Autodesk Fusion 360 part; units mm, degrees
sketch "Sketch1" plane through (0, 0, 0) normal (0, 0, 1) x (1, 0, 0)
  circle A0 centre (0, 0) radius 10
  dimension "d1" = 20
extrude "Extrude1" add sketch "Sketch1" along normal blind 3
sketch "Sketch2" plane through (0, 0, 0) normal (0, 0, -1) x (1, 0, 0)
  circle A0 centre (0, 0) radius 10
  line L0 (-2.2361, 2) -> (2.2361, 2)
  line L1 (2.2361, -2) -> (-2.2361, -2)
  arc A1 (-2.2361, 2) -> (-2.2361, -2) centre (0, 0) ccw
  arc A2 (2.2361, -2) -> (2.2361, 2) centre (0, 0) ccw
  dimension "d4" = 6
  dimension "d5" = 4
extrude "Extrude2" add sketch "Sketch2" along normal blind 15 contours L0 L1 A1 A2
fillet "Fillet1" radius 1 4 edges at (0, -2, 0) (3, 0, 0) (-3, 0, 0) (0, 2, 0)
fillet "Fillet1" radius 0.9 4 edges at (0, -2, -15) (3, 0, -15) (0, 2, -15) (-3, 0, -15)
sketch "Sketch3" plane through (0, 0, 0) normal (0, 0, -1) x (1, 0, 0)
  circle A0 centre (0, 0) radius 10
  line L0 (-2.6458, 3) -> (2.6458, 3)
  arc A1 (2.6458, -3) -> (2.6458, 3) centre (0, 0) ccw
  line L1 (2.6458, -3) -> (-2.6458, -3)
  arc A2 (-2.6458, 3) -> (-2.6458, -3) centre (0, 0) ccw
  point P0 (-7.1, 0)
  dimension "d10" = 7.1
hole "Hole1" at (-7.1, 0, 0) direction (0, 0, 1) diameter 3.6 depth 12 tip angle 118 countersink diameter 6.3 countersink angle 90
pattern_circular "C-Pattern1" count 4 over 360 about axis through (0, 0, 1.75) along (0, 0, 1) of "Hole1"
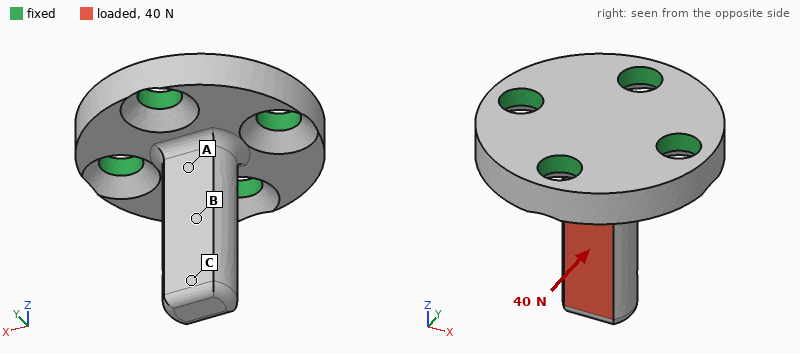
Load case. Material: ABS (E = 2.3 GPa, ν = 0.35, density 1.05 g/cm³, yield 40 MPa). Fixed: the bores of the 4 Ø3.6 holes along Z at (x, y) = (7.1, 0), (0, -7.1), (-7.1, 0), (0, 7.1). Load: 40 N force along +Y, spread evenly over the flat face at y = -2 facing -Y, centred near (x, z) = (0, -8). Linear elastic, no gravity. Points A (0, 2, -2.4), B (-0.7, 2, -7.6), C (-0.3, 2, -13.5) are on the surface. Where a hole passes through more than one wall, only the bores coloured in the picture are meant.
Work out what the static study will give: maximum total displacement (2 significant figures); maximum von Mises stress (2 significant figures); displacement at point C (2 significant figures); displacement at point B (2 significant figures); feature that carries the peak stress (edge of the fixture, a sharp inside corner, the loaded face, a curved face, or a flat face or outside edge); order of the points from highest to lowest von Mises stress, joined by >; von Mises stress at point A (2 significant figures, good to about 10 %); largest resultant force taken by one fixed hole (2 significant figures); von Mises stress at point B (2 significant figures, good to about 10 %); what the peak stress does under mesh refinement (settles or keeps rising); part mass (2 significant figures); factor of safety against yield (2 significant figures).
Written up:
0.34 mm
30 MPa
0.31 mm
0.15 mm
a curved face
A > B > C
14 MPa
37 N
4.9 MPa
settles
1.2 g
1.3
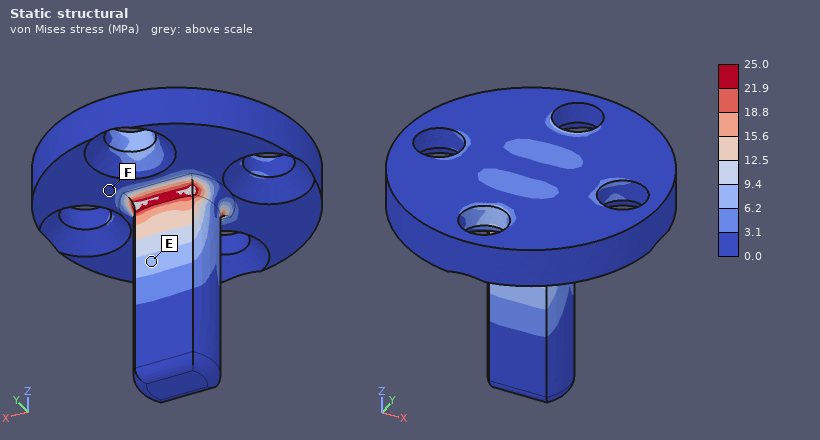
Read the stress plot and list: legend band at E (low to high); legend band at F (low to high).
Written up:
6.2 to 9.4 MPa
0.0 to 3.1 MPa
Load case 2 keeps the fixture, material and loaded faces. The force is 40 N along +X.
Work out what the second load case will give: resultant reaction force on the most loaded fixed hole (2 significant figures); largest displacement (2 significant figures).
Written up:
38 N
0.21 mm
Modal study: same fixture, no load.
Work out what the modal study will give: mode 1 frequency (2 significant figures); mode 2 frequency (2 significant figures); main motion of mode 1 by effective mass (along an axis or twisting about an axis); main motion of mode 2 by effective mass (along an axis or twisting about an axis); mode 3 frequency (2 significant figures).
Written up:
3600 Hz
4800 Hz
along Y
along X
14 kHz
